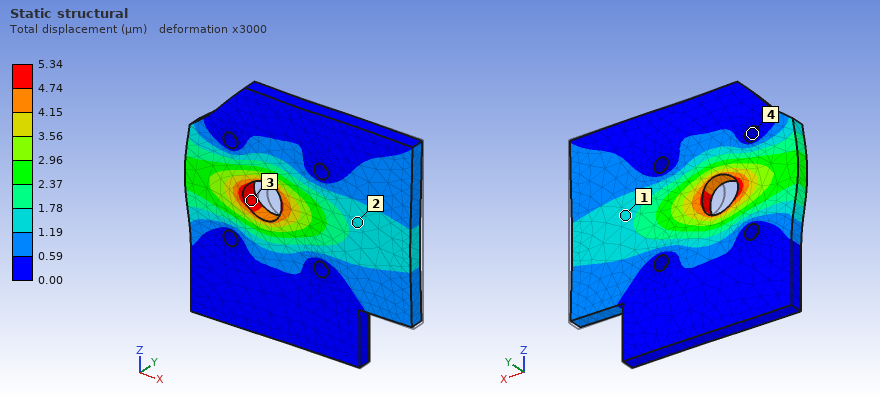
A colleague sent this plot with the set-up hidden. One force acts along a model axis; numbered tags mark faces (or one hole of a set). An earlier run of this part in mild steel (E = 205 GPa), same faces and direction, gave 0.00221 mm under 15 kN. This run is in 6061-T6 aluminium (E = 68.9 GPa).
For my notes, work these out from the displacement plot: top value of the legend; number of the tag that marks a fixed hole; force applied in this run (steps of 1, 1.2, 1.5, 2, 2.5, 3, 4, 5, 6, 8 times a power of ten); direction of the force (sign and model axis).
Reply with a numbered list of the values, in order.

1. 5.34 µm
2. 4
3. 12 kN
4. -X
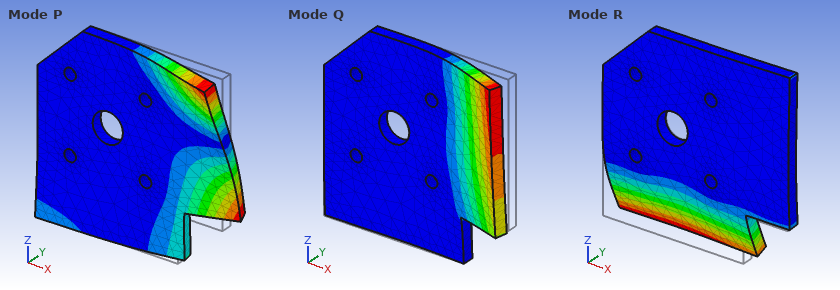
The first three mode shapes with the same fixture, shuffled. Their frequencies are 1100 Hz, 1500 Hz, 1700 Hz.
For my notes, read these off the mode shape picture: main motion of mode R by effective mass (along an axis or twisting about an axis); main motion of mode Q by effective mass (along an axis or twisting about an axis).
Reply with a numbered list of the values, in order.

1. along Y
2. along Y
